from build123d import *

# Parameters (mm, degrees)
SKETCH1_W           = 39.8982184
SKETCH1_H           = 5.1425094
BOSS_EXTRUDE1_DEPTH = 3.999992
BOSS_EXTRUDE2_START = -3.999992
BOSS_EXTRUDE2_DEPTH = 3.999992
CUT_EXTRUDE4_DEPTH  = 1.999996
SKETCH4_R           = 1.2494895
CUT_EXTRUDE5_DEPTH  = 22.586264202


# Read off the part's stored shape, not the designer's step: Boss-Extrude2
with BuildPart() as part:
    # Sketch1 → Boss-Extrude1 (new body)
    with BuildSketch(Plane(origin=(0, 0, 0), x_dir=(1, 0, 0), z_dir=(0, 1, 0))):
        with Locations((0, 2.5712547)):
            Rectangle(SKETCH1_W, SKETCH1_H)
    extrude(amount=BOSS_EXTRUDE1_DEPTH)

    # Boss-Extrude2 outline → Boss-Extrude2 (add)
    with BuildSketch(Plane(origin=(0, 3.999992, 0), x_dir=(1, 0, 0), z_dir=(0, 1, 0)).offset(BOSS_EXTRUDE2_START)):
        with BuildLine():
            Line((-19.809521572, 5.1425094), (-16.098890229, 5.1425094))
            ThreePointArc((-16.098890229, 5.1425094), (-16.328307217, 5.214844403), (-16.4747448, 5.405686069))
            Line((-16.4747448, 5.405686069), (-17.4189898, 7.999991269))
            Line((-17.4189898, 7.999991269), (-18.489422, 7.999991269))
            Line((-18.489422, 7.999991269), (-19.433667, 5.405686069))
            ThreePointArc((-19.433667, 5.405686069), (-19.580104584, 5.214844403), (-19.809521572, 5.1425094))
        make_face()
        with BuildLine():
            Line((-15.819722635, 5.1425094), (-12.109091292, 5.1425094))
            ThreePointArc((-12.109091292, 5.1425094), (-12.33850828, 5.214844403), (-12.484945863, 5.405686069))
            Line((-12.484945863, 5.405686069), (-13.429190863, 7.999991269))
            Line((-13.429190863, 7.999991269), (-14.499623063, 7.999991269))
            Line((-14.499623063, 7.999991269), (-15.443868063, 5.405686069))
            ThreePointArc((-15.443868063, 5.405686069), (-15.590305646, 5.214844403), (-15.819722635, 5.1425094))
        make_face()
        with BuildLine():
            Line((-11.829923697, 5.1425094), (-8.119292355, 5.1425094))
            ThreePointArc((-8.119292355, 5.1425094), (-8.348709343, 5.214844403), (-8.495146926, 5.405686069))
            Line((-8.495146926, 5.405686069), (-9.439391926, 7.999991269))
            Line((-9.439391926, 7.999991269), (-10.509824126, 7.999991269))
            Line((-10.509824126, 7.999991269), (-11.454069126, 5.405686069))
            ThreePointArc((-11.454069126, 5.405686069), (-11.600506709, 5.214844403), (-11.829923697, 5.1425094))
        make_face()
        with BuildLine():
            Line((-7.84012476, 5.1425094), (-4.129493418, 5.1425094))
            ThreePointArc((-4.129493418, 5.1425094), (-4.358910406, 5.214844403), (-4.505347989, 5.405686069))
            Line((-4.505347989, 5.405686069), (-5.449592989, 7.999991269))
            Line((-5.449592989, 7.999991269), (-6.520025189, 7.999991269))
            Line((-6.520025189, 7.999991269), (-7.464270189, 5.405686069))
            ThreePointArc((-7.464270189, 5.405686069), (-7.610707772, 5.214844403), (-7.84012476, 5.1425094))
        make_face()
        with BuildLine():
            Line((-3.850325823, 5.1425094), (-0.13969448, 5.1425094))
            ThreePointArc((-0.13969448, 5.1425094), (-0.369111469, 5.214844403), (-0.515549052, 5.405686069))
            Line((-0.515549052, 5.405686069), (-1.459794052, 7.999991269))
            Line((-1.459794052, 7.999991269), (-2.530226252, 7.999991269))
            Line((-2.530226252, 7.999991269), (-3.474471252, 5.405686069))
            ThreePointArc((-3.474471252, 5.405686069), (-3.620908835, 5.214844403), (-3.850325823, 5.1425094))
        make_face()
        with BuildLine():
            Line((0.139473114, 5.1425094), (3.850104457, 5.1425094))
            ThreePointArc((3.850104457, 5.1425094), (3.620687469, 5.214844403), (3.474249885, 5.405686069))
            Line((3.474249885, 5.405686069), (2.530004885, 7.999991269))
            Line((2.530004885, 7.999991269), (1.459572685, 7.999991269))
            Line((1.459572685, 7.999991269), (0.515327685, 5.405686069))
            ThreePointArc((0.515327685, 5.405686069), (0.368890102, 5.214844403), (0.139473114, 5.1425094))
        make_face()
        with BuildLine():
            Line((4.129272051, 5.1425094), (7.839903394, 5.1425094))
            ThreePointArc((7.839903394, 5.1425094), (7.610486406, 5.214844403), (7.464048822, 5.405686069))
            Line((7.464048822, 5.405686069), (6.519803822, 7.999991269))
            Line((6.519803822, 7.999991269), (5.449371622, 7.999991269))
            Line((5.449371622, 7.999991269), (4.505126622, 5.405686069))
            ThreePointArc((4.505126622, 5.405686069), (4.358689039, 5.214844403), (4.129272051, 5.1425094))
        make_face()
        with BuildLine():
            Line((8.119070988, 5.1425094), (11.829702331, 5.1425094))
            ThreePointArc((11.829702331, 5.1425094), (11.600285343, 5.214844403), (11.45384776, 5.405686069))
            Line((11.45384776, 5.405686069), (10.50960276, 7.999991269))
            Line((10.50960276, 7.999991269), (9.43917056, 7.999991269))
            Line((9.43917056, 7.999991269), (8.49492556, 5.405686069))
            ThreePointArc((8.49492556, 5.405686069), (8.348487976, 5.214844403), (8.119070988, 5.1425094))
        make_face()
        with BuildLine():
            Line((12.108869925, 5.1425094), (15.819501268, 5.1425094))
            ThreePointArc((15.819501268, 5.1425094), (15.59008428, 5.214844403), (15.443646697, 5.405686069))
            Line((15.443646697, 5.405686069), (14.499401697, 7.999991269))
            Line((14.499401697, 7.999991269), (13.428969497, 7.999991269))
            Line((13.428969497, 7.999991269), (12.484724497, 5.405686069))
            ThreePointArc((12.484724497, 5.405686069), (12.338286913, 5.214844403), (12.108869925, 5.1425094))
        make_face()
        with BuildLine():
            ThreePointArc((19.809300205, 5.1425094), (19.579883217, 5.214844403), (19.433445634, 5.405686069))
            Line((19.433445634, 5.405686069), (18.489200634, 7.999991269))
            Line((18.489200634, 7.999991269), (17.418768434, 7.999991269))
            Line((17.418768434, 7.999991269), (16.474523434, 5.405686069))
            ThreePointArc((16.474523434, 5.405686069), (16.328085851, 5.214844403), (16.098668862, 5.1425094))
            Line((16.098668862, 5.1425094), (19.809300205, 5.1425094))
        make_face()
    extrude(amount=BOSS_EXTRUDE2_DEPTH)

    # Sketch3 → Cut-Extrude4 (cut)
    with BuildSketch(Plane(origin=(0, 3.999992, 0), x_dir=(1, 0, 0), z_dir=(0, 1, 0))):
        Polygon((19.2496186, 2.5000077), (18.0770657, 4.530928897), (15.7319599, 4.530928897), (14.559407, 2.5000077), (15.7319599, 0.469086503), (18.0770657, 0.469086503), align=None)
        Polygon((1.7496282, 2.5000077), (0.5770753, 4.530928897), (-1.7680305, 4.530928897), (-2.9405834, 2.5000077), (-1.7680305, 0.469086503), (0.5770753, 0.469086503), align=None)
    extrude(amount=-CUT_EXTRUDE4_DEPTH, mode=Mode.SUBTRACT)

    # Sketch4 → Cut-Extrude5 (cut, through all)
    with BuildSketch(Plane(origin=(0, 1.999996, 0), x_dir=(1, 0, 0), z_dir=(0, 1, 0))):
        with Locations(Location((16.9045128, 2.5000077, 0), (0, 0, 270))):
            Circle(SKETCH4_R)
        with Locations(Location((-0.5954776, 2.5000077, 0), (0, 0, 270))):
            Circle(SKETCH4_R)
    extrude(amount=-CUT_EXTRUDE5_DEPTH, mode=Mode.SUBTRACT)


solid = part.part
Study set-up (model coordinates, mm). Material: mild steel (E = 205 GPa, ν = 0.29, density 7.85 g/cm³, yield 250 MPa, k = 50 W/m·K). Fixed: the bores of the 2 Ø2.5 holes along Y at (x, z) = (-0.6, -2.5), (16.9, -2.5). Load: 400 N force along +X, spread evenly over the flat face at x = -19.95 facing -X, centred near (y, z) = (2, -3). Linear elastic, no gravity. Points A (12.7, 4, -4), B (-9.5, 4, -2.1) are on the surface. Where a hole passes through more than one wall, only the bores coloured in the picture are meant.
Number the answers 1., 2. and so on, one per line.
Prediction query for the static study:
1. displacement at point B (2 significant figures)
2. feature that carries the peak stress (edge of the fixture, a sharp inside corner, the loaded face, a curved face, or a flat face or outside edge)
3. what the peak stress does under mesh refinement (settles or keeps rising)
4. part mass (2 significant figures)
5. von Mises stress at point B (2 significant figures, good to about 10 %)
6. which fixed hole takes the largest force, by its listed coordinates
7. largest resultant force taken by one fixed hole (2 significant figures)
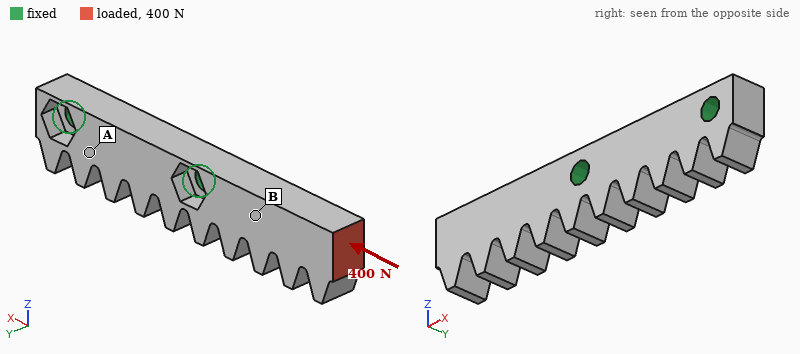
1. 3.5 µm
2. edge of the fixture
3. keeps rising
4. 7.7 g
5. 19 MPa
6. (-0.6, -2.5)
7. 360 N
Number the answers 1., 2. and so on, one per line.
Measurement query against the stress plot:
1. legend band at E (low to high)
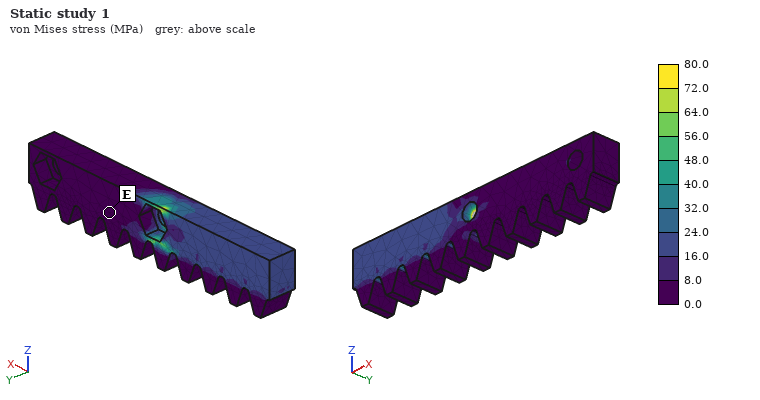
1. 0.0 to 8.0 MPa
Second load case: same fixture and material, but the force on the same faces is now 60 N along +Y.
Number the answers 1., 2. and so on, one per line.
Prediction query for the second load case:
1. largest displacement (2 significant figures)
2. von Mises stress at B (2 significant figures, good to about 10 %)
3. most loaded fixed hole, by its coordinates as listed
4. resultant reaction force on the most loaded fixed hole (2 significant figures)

1. 39 µm
2. 44 MPa
3. (-0.6, -2.5)
4. 100 N
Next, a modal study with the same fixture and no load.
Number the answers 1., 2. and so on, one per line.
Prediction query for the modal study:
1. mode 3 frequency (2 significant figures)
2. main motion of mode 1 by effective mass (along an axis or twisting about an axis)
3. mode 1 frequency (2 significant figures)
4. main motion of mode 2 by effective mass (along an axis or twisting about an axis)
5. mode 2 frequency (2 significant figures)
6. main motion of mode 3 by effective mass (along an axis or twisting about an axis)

1. 24 kHz
2. along Y
3. 6000 Hz
4. along Z
5. 8500 Hz
6. twisting about X
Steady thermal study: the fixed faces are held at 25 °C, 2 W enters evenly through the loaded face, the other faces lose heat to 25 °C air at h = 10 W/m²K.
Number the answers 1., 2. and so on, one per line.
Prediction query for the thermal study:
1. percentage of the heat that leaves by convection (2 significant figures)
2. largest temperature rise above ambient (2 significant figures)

1. 4.5 %
2. 35 K
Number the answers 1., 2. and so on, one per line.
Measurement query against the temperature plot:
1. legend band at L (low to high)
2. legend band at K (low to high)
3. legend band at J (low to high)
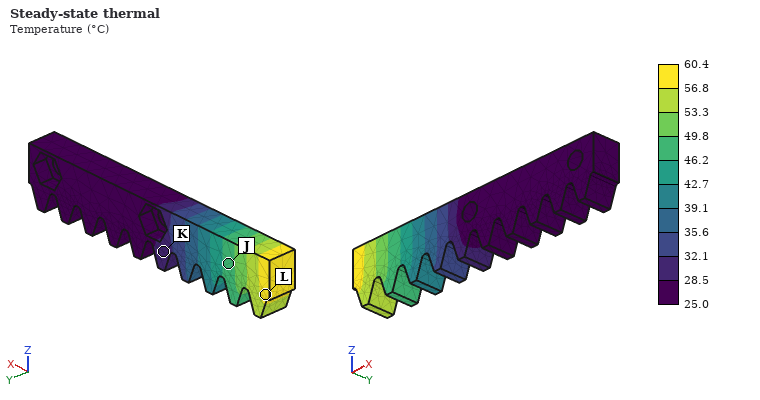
1. 56.8 to 60.4 °C
2. 28.5 to 32.1 °C
3. 46.2 to 49.8 °C
